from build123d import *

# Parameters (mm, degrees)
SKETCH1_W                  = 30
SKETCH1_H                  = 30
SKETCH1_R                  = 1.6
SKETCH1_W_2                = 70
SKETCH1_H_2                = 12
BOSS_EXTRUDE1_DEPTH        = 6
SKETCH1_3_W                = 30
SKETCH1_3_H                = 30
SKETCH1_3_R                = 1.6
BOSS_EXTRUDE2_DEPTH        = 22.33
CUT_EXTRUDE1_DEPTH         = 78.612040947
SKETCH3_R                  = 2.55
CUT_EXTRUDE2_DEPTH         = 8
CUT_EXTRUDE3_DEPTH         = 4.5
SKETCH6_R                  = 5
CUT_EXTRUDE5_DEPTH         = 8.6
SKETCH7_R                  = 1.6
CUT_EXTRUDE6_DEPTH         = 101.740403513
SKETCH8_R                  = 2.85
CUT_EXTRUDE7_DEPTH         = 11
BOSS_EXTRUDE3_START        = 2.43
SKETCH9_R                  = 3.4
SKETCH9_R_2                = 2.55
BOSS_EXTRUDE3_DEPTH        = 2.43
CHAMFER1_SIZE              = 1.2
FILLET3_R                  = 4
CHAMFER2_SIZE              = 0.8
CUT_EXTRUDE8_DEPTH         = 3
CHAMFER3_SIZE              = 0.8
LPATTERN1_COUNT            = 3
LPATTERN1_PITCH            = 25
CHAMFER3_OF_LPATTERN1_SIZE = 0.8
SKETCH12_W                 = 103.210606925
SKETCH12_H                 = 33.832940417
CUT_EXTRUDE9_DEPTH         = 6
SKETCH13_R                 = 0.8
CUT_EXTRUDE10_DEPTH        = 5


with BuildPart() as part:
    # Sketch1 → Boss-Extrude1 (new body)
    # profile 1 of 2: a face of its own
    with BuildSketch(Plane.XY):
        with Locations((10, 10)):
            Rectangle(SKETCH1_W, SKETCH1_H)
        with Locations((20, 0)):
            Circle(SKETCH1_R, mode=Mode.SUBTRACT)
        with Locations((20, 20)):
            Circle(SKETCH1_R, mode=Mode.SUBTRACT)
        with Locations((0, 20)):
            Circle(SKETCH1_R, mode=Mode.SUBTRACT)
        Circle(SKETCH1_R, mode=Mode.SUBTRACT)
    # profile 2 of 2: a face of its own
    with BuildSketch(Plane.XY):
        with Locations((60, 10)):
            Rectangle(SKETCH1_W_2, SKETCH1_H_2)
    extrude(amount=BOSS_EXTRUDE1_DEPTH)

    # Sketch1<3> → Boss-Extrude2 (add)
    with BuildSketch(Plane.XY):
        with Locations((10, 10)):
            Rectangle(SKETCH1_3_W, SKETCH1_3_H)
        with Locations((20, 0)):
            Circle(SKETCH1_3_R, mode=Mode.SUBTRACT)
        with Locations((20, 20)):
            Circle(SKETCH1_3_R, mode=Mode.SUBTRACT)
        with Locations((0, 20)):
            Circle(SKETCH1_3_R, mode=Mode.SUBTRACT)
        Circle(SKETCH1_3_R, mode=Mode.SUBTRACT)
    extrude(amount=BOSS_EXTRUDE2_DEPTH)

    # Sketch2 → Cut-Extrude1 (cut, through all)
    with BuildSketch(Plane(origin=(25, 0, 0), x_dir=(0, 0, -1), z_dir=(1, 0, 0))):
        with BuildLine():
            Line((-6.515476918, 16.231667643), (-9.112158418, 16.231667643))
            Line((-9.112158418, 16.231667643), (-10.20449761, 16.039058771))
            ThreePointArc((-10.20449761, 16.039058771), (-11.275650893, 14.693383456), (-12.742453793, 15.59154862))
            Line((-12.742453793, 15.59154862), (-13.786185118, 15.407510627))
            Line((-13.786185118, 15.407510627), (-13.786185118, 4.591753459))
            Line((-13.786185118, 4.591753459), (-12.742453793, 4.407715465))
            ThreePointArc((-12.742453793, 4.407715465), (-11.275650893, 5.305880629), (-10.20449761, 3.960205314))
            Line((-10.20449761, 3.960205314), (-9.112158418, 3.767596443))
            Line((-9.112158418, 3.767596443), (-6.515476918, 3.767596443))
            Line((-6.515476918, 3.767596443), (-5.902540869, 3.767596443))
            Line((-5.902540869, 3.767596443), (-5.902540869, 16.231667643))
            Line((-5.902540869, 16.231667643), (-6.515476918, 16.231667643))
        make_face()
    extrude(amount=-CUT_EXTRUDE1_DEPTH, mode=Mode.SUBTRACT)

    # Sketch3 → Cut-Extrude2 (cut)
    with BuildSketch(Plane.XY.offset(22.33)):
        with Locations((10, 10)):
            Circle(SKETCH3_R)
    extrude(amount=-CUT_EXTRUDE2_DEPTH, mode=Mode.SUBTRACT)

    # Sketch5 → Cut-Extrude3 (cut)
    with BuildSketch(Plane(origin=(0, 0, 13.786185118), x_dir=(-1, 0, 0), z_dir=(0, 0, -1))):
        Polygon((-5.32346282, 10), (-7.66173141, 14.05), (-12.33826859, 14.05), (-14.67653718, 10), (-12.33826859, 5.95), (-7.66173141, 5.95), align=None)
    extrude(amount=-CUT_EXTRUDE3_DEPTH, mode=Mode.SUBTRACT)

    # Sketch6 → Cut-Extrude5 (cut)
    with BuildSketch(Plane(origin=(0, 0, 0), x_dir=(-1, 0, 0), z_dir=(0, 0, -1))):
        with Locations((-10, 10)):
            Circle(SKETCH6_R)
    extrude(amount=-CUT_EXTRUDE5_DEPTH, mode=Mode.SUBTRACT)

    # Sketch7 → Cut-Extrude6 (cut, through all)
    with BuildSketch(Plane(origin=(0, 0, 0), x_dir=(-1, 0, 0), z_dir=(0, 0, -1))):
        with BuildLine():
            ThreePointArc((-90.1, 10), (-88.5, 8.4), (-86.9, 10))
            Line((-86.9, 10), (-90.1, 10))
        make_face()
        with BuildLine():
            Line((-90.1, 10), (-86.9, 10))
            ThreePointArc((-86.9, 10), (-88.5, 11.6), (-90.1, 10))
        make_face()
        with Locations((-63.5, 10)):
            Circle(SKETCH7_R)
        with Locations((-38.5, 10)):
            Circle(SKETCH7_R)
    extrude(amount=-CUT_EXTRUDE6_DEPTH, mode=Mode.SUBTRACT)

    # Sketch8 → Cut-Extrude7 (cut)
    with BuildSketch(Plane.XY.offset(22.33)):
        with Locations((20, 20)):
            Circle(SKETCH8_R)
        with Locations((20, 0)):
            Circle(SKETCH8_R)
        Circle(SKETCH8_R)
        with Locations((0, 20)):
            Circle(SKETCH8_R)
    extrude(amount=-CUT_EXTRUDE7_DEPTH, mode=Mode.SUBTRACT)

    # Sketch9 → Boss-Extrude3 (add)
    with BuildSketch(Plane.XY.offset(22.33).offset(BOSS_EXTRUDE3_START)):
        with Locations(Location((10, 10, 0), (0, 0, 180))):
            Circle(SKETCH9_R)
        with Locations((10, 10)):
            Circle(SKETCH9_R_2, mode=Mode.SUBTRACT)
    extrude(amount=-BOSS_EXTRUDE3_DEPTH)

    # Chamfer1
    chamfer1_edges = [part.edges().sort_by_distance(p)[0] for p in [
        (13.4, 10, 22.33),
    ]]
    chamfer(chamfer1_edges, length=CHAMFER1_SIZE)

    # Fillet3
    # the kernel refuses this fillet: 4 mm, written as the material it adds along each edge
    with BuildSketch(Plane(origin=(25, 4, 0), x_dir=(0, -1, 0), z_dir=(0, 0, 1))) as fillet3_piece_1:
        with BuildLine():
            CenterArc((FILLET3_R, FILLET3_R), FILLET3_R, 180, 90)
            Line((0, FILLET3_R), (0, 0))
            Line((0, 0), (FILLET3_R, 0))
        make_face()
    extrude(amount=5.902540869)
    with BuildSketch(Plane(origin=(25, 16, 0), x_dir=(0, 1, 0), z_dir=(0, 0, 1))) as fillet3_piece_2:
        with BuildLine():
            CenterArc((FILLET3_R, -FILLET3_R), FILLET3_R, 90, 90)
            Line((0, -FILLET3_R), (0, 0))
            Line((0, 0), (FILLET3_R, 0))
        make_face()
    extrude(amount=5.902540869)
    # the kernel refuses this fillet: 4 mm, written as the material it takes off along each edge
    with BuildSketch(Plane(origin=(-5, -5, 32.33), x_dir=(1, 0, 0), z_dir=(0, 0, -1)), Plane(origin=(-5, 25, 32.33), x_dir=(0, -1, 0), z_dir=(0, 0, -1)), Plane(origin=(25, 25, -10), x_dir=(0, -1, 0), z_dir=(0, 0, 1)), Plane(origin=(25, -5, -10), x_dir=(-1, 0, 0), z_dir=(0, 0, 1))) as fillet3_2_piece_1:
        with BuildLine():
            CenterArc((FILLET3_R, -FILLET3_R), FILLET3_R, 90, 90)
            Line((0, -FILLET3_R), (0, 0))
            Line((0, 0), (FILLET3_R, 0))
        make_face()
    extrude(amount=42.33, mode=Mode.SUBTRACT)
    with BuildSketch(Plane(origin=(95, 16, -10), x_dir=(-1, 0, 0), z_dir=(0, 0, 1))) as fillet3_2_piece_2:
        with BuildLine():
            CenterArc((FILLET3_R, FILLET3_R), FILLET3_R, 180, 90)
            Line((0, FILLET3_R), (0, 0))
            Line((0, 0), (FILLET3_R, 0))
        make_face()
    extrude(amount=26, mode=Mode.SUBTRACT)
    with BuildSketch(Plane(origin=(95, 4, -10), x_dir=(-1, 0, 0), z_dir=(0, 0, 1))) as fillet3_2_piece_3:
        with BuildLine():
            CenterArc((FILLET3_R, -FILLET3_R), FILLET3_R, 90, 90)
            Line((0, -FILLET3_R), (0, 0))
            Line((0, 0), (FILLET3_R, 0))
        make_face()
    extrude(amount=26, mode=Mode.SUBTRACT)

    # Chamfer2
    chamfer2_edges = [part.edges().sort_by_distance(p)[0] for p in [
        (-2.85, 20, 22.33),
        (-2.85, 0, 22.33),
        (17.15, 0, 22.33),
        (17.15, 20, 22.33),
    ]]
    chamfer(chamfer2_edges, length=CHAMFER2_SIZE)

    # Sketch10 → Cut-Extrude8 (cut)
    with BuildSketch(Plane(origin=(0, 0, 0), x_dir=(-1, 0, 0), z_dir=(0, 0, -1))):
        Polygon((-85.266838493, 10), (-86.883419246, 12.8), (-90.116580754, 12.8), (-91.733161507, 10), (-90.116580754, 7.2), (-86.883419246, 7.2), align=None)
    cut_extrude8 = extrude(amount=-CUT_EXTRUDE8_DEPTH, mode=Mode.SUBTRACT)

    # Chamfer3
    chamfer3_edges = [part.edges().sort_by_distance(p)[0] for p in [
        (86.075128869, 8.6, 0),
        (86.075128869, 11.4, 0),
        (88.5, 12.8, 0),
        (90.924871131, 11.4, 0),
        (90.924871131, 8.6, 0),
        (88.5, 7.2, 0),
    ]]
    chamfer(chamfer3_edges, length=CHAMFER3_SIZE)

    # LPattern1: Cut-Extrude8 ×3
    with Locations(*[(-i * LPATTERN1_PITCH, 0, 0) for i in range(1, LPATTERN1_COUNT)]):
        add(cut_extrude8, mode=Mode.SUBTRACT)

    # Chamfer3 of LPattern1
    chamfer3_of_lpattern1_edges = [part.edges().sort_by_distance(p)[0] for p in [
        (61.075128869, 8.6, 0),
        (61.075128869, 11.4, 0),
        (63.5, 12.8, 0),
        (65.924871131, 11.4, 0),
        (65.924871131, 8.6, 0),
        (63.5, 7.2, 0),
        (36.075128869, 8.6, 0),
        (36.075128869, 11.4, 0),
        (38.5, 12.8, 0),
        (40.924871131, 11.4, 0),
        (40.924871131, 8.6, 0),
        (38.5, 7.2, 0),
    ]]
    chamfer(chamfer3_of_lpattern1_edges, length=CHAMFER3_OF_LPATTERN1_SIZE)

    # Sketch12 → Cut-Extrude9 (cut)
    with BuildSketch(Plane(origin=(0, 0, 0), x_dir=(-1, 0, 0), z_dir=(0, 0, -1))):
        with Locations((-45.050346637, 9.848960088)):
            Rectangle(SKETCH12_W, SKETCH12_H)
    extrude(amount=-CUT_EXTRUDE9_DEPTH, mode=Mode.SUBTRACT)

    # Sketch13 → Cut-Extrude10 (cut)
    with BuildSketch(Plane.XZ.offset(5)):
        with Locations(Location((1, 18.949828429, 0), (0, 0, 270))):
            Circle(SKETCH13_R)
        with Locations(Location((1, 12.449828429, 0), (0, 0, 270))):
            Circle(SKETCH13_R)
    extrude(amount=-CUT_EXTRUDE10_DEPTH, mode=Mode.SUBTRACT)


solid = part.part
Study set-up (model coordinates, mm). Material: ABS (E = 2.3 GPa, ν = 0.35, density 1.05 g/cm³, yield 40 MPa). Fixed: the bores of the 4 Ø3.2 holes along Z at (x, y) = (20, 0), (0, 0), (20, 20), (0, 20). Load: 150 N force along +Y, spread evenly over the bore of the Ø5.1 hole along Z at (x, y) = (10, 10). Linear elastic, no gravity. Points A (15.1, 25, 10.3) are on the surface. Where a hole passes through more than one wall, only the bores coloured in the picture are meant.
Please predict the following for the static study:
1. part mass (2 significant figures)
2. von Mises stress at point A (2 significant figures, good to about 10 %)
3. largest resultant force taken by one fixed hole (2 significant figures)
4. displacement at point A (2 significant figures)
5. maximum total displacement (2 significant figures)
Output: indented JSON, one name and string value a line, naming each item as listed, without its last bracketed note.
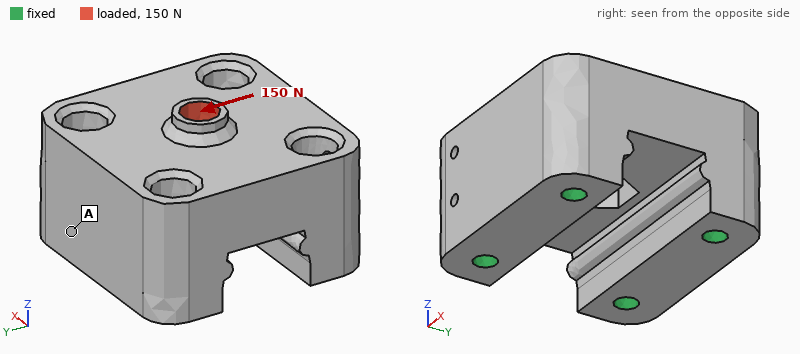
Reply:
{
  "part mass": "11 g",
  "von Mises stress at point A": "0.54 MPa",
  "largest resultant force taken by one fixed hole": "53 N",
  "displacement at point A": "6.9 µm",
  "maximum total displacement": "28 µm"
}
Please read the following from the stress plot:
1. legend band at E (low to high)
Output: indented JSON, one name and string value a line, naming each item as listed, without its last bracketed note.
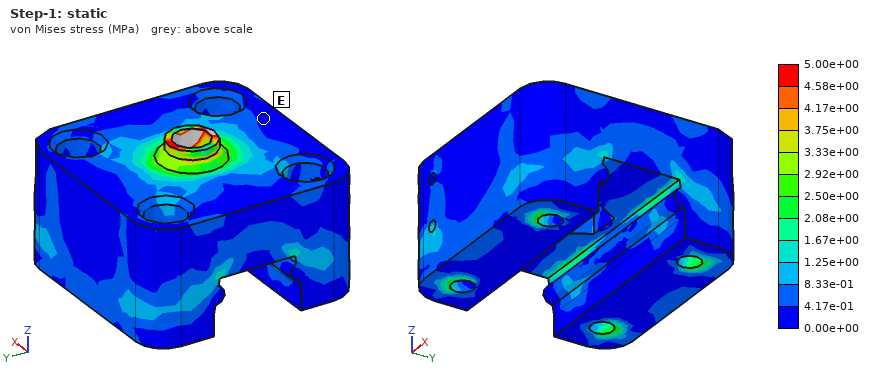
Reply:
{
  "legend band at E": "0.00e+00 to 4.17e-01 MPa"
}
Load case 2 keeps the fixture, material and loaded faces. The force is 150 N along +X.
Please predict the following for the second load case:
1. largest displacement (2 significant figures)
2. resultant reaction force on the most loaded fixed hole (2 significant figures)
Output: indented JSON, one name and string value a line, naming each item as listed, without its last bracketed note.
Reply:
{
  "largest displacement": "26 µm",
  "resultant reaction force on the most loaded fixed hole": "58 N"
}
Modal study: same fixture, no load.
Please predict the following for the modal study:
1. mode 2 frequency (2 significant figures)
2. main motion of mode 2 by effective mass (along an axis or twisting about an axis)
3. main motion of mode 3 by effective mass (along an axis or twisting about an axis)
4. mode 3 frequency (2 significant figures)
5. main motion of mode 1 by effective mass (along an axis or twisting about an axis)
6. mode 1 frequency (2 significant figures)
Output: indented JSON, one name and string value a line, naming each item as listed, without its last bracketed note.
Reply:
{
  "mode 2 frequency": "8900 Hz",
  "main motion of mode 2 by effective mass": "along X",
  "main motion of mode 3 by effective mass": "twisting about Z",
  "mode 3 frequency": "11 kHz",
  "main motion of mode 1 by effective mass": "along Y",
  "mode 1 frequency": "7200 Hz"
}
